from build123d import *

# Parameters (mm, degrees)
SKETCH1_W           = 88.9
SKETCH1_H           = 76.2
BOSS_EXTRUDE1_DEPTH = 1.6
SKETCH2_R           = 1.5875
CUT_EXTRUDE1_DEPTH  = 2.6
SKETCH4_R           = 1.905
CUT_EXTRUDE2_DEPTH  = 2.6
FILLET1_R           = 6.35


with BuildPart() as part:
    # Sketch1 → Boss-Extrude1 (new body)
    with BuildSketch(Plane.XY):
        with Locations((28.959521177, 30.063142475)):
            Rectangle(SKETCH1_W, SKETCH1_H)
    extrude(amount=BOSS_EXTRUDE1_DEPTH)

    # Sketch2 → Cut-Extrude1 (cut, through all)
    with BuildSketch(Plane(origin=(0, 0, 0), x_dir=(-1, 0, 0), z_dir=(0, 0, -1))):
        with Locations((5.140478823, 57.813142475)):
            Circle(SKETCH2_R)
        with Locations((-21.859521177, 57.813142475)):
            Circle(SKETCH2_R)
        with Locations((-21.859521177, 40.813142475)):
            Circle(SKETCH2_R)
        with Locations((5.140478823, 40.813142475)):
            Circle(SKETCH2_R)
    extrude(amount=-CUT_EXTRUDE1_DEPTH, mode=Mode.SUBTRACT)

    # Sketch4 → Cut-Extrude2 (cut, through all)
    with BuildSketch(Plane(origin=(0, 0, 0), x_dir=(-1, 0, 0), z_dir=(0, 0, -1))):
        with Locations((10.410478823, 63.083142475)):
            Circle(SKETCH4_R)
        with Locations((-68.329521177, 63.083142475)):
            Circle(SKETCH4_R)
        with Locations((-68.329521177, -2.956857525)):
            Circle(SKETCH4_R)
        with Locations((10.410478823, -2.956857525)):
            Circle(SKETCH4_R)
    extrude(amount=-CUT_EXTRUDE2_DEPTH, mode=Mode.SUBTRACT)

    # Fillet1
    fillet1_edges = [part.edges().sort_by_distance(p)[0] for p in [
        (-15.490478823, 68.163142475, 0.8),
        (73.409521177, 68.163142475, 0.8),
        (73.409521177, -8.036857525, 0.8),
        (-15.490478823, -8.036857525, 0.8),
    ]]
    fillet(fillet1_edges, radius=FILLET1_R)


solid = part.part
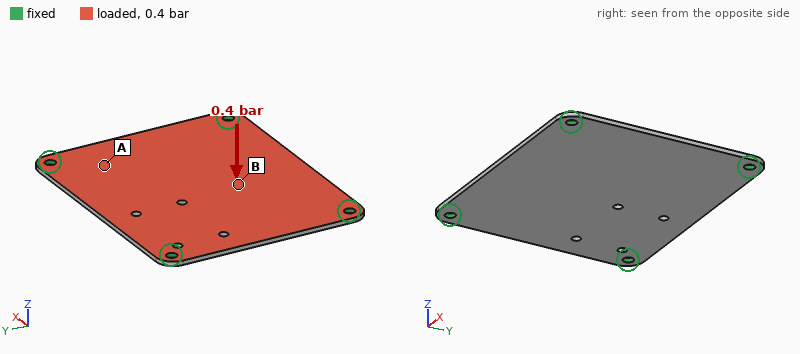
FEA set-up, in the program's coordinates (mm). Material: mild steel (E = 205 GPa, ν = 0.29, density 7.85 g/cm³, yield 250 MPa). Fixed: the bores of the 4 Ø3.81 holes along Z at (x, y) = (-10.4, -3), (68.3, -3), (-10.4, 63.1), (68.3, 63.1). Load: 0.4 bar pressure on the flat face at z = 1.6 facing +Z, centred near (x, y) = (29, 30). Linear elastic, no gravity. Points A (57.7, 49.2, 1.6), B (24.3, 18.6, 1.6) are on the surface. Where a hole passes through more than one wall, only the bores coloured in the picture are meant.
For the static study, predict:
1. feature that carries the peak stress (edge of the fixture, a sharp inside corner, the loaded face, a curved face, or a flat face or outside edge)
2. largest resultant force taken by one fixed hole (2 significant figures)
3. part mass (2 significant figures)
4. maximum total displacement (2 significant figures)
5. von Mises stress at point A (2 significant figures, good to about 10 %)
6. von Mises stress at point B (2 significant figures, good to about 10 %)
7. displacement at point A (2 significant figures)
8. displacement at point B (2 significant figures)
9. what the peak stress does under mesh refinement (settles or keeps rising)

edge of the fixture
67 N
84 g
0.11 mm
11 MPa
26 MPa
0.045 mm
0.11 mm
keeps rising
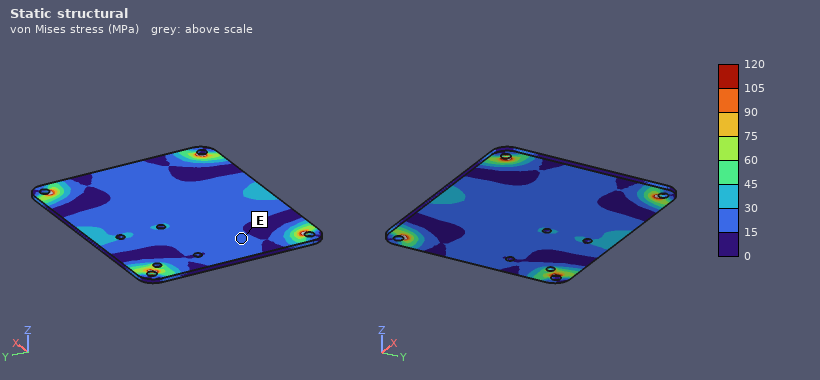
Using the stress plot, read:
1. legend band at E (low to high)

15 to 30 MPa
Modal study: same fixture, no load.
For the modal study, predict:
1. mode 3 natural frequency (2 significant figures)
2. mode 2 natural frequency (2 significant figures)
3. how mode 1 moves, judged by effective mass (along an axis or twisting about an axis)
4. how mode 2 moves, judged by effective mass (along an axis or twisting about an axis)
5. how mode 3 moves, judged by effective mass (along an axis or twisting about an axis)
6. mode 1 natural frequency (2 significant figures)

2000 Hz
1600 Hz
along Z
twisting about X
twisting about Y
1000 Hz
